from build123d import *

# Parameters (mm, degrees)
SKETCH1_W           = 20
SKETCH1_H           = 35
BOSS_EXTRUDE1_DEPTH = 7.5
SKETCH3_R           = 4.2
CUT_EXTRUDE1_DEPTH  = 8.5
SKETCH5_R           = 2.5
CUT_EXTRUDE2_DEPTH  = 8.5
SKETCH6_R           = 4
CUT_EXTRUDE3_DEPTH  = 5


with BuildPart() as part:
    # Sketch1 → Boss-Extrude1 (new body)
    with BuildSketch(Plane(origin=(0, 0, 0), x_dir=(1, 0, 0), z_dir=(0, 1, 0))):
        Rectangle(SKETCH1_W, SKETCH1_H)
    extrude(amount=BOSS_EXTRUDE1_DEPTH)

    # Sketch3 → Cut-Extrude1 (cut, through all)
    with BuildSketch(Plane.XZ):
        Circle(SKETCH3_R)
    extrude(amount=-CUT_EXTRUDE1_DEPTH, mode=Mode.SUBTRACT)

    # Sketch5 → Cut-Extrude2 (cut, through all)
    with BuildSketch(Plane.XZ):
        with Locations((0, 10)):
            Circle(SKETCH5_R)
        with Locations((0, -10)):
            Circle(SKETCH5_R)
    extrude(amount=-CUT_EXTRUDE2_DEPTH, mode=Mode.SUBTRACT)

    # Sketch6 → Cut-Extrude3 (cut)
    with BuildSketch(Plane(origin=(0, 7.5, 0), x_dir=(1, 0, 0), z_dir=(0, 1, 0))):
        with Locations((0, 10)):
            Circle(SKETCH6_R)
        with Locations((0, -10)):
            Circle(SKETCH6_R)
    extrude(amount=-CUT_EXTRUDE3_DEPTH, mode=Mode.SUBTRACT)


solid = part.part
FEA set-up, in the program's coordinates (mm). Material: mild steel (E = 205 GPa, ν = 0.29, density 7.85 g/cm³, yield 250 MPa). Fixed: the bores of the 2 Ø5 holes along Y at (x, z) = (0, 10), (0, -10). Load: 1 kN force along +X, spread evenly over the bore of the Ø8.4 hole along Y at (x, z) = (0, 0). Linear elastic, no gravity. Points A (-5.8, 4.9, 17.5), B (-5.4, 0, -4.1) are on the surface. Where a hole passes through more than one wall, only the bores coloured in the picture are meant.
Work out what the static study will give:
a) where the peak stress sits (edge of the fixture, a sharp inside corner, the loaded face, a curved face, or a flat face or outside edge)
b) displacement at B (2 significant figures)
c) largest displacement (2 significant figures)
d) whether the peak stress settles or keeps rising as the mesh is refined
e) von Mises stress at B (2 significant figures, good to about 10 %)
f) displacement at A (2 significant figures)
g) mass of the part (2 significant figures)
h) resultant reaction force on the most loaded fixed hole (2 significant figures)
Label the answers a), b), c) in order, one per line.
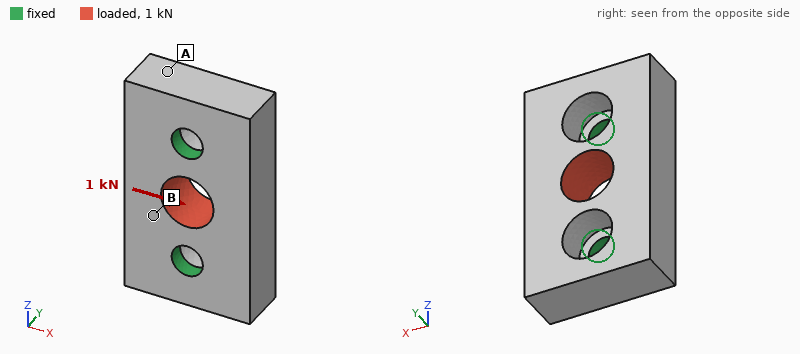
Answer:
a) edge of the fixture
b) 1.0 µm
c) 2.9 µm
d) keeps rising
e) 10.0 MPa
f) 1.1 µm
g) 33 g
h) 500 N
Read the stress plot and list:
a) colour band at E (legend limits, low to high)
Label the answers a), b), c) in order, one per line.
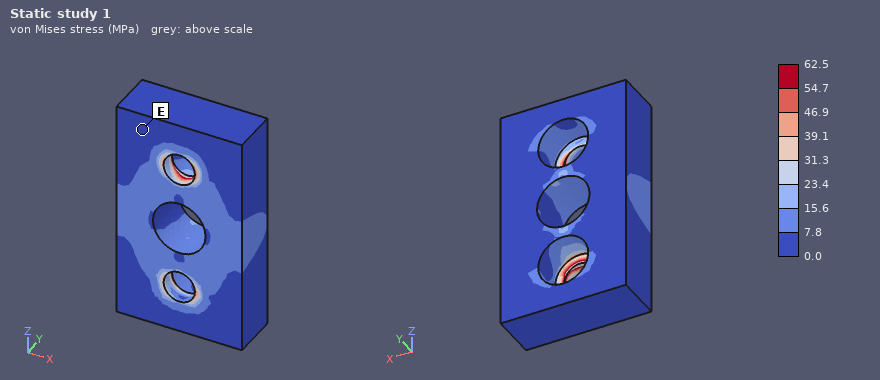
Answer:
a) 0.0 to 7.8 MPa
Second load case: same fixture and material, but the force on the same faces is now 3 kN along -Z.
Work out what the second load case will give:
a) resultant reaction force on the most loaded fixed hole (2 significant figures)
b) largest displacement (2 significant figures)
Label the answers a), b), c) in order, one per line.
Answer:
a) 1.5 kN
b) 2.7 µm
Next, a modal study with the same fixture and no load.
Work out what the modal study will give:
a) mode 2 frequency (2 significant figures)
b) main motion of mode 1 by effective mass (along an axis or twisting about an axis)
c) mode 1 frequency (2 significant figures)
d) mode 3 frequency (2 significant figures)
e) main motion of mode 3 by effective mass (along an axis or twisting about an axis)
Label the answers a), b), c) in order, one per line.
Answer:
a) 25 kHz
b) along X
c) 15 kHz
d) 31 kHz
e) along Z
